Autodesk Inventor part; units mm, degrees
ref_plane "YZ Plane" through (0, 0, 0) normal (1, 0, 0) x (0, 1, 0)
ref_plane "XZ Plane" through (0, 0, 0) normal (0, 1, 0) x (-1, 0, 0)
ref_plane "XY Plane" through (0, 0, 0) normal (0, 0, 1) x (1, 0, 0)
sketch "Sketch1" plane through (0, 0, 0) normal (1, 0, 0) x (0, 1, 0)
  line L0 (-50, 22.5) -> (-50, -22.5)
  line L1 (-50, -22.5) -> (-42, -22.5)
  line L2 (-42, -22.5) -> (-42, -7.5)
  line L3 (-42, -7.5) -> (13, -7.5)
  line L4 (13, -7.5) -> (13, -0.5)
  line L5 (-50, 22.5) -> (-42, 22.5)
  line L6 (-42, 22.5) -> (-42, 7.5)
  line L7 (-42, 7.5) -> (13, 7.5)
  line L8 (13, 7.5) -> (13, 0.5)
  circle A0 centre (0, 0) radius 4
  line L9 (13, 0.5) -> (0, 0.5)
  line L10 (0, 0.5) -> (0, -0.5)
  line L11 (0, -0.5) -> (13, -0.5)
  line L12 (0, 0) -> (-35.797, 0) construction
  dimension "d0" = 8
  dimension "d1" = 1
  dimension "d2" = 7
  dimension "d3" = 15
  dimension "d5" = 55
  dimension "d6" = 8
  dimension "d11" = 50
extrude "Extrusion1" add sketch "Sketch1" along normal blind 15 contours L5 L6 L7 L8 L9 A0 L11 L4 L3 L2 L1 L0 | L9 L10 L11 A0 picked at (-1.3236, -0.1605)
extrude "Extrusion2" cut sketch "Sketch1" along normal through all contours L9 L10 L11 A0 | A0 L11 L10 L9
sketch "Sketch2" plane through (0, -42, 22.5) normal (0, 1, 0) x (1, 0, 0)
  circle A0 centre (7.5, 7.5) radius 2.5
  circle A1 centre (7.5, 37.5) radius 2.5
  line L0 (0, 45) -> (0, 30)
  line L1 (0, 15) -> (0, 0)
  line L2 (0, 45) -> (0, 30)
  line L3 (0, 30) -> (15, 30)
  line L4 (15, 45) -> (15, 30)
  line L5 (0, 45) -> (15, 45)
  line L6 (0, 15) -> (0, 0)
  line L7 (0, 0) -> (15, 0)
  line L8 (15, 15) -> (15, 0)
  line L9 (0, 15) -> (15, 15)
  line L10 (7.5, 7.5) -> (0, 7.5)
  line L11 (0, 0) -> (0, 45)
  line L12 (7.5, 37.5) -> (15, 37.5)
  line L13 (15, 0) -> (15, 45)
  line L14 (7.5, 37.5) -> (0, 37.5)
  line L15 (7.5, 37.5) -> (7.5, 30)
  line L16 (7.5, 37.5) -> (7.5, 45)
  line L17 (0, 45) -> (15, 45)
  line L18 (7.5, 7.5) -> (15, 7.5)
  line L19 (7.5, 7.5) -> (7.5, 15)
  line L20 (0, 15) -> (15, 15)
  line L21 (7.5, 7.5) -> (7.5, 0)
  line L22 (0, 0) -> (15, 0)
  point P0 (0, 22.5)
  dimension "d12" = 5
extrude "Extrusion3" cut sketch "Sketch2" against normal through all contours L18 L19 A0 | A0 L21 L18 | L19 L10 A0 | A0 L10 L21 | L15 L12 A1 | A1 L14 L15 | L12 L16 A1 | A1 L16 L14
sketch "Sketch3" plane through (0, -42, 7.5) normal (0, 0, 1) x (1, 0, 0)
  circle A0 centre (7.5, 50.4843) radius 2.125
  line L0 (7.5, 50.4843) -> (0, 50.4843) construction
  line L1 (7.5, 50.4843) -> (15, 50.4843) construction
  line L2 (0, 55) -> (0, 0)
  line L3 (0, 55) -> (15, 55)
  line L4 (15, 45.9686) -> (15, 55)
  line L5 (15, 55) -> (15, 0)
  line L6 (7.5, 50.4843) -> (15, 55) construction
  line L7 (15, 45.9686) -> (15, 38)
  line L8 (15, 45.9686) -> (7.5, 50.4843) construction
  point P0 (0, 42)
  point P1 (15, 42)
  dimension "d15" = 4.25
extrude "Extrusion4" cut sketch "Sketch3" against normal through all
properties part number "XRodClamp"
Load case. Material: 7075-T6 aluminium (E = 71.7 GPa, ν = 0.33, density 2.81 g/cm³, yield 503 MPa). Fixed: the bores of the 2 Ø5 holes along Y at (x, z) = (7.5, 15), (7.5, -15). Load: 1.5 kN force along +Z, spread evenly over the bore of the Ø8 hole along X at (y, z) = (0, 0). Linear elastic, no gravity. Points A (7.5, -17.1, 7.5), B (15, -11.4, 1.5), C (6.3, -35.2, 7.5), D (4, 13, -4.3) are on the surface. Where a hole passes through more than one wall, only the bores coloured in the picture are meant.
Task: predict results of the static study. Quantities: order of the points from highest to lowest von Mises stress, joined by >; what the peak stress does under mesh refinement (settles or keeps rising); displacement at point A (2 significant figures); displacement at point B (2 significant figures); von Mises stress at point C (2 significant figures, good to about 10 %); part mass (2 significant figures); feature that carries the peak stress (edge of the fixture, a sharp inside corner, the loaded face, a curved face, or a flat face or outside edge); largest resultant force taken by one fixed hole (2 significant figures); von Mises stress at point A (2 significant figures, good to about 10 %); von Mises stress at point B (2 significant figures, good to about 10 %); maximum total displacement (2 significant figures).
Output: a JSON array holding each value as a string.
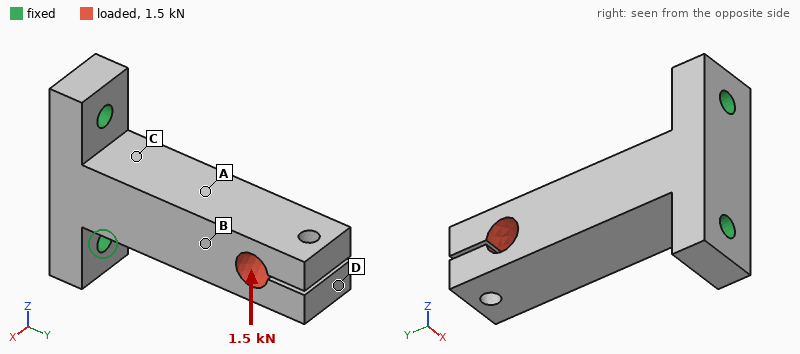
["C > A > B > D", "keeps rising", "0.11 mm", "0.13 mm", "95 MPa", "46 g", "a sharp inside corner", "3.1 kN", "45 MPa", "21 MPa", "0.31 mm"]
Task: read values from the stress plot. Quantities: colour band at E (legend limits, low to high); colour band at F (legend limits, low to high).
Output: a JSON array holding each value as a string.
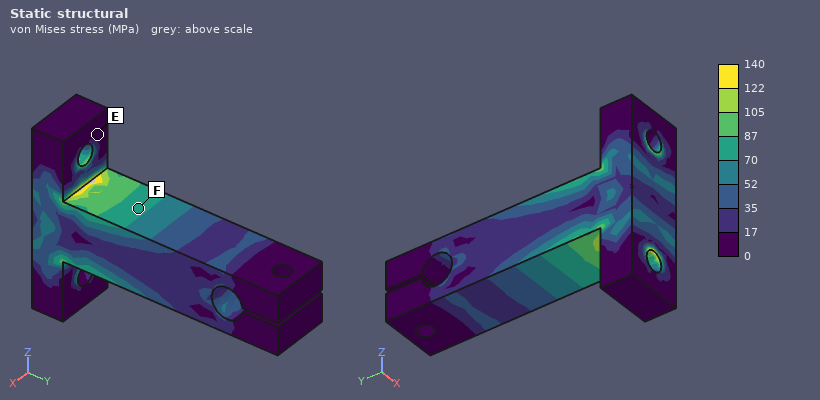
["0 to 17 MPa", "70 to 87 MPa"]
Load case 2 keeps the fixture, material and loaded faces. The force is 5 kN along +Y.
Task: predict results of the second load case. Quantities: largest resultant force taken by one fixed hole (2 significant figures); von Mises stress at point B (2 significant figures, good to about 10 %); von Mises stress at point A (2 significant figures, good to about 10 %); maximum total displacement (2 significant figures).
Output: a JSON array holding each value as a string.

["2.6 kN", "29 MPa", "22 MPa", "95 µm"]
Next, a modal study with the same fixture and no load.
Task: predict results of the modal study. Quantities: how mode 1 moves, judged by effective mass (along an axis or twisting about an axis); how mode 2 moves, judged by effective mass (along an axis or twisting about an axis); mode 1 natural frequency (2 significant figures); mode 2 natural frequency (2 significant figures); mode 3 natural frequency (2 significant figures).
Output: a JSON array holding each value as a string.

["along X", "along Z", "2300 Hz", "3300 Hz", "7500 Hz"]
